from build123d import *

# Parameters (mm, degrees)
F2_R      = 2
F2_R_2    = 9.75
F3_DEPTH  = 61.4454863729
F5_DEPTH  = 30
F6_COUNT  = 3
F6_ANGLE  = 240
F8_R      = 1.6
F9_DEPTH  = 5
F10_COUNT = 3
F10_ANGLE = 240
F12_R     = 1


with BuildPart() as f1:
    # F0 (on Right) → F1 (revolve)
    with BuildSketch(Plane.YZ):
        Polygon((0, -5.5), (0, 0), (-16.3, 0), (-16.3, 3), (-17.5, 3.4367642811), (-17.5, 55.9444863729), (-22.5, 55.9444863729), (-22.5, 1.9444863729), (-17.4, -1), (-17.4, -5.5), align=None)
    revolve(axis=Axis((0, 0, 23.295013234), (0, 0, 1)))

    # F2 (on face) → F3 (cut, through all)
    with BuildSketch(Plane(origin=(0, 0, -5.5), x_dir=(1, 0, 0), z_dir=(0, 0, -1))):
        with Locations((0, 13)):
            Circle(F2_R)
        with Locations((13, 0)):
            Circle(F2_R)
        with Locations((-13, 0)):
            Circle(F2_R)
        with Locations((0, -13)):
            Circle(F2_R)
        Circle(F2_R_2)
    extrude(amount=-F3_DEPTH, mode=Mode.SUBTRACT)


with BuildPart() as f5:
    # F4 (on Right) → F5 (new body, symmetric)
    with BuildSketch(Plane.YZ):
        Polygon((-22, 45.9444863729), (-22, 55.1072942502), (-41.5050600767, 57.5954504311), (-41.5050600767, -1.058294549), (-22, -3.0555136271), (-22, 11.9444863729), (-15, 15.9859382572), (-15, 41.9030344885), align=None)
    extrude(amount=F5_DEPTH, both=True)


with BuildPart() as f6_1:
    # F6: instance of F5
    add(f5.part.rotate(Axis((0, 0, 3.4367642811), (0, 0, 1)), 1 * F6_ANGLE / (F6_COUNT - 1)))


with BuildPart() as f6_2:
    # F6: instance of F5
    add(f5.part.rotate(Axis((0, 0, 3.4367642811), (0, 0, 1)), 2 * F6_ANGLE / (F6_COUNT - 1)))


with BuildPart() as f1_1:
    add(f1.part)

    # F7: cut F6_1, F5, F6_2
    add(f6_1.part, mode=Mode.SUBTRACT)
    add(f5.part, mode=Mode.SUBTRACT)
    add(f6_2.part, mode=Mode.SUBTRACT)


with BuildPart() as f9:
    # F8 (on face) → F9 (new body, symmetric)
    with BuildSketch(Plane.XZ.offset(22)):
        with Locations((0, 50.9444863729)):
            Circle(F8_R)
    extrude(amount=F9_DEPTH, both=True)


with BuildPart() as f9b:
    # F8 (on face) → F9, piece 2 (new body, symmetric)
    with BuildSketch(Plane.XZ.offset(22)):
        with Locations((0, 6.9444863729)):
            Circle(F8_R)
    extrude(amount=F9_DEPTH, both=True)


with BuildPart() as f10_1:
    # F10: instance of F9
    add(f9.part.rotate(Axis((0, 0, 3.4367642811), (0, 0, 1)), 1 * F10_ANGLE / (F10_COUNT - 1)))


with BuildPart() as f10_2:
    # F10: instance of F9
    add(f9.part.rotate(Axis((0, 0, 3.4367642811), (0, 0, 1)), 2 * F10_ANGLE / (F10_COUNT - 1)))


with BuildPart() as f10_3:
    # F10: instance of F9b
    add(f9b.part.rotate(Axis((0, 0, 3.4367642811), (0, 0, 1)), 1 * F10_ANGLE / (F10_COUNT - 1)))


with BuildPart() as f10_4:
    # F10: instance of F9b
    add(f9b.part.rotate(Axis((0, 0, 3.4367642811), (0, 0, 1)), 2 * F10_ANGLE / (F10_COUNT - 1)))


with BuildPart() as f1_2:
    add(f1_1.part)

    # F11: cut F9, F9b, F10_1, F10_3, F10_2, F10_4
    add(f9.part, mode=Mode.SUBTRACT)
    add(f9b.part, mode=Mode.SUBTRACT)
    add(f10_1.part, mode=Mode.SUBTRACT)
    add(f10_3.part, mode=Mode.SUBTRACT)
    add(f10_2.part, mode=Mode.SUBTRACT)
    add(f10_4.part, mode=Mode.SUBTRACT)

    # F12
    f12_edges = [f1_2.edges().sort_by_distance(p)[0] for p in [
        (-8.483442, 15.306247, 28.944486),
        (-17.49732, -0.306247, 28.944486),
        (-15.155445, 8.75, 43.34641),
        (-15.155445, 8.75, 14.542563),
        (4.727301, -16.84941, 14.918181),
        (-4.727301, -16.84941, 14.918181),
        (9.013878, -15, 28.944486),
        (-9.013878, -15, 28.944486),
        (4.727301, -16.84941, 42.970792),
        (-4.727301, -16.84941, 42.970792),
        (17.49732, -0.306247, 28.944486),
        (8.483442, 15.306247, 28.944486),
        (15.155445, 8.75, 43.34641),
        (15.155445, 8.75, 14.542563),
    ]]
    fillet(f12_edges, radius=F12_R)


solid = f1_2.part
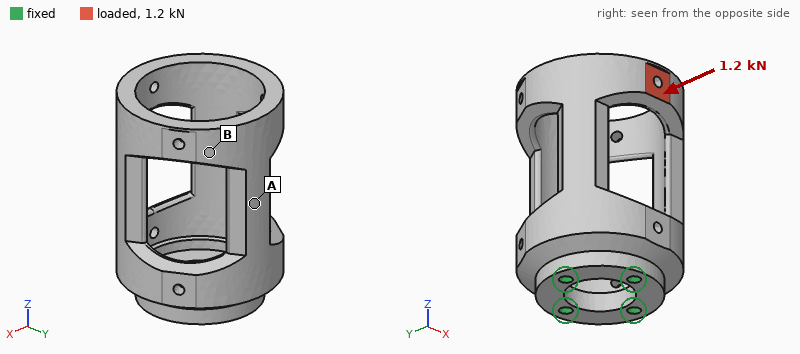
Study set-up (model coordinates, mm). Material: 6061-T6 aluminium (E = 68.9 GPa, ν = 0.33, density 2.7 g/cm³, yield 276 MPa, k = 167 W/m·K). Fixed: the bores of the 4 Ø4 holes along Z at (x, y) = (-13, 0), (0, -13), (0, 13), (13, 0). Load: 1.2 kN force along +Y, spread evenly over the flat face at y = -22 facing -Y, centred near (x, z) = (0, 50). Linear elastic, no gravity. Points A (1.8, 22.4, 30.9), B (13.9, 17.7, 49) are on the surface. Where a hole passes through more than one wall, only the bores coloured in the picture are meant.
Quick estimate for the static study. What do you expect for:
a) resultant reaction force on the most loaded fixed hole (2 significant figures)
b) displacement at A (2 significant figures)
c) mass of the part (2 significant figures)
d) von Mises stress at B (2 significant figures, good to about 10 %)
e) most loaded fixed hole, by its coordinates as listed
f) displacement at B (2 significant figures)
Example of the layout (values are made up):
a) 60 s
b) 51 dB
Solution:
a) 2.0 kN
b) 0.080 mm
c) 67 g
d) 31 MPa
e) (0, -13)
f) 0.13 mm
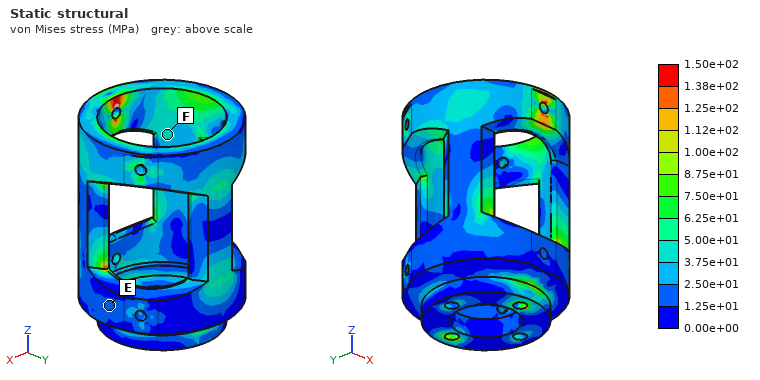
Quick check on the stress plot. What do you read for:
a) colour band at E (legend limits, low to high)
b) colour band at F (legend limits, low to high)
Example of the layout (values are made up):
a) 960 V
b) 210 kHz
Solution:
a) 1.25e+01 to 2.50e+01 MPa
b) 3.75e+01 to 5.00e+01 MPa
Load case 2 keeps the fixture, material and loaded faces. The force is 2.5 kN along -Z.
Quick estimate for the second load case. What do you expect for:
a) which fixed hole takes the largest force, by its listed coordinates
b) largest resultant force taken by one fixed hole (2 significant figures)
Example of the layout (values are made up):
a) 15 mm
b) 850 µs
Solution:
a) (0, -13)
b) 1.8 kN
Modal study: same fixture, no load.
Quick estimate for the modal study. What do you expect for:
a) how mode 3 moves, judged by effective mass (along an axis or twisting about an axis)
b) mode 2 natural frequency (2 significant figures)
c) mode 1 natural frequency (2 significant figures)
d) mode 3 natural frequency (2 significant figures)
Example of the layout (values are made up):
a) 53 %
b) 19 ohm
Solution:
a) twisting about Z
b) 2800 Hz
c) 2800 Hz
d) 5500 Hz
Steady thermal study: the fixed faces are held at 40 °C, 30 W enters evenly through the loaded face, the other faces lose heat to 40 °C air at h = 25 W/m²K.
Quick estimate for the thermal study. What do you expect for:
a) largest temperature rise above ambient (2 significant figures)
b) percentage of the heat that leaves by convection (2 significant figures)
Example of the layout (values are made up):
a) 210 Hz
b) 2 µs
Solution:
a) 66 K
b) 20 %
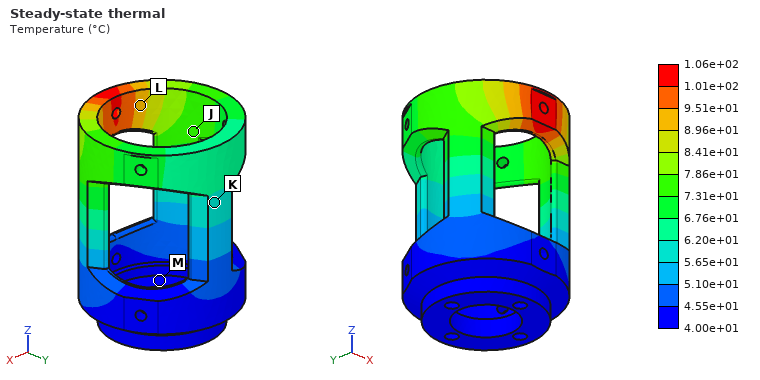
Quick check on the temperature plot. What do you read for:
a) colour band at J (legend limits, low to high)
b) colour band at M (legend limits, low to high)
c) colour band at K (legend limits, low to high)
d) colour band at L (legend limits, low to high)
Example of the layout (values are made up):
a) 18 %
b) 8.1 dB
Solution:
a) 7.31e+01 to 7.86e+01 °C
b) 4.00e+01 to 4.55e+01 °C
c) 5.65e+01 to 6.20e+01 °C
d) 8.96e+01 to 9.51e+01 °C
